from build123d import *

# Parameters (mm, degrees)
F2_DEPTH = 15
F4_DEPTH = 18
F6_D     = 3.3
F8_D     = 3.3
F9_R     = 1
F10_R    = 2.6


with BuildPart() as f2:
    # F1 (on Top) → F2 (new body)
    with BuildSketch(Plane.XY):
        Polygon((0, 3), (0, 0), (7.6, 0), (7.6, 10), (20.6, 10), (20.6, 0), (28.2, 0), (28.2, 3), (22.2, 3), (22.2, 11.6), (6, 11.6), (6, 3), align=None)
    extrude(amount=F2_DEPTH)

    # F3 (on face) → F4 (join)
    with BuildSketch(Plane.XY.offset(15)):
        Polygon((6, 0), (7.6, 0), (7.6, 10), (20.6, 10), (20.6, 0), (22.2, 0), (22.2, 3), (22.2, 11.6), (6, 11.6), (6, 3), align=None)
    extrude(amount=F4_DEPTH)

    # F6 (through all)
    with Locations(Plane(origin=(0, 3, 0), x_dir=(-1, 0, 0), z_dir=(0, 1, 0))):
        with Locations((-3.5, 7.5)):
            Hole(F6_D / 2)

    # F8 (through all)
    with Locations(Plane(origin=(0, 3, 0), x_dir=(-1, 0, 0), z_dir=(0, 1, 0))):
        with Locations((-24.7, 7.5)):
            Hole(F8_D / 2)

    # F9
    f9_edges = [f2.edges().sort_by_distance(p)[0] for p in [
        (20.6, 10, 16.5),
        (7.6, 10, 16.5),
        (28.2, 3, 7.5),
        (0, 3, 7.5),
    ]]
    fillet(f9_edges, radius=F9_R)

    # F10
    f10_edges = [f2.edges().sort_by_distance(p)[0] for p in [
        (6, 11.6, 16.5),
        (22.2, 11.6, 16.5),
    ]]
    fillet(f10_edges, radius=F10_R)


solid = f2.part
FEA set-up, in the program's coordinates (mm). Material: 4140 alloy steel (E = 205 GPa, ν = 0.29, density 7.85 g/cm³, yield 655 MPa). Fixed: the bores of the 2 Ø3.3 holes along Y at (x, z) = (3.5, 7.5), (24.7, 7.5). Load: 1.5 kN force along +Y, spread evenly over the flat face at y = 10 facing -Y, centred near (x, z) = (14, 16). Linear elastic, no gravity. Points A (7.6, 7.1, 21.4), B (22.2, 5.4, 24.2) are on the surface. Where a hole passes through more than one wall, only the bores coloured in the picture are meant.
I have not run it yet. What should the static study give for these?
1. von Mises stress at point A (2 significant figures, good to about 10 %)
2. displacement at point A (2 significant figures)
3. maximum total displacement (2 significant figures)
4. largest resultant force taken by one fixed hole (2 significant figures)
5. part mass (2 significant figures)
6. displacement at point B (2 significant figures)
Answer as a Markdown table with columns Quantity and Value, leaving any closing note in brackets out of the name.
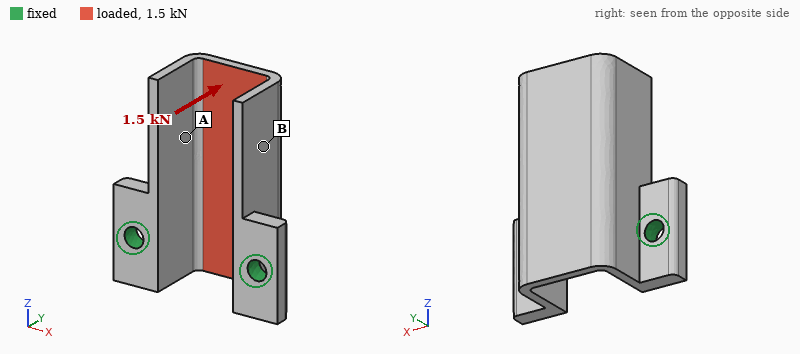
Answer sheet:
| Quantity | Value |
|---|---|
| von Mises stress at point A | 98 MPa |
| displacement at point A | 0.044 mm |
| maximum total displacement | 0.10 mm |
| largest resultant force taken by one fixed hole | 800 N |
| part mass | 18 g |
| displacement at point B | 0.049 mm |
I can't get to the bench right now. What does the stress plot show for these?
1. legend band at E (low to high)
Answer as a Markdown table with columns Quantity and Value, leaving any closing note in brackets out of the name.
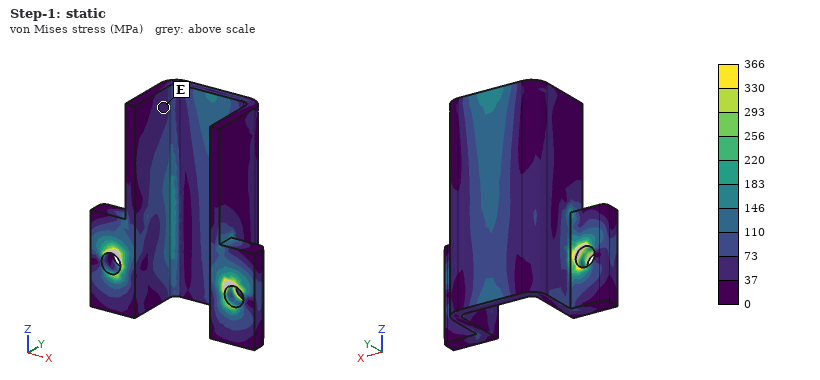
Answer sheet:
| Quantity | Value |
|---|---|
| legend band at E | 37 to 73 MPa |
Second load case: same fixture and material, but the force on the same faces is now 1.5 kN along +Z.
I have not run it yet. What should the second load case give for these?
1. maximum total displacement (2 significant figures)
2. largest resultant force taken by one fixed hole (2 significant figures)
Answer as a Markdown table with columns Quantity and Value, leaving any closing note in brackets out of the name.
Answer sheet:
| Quantity | Value |
|---|---|
| maximum total displacement | 69 µm |
| largest resultant force taken by one fixed hole | 750 N |
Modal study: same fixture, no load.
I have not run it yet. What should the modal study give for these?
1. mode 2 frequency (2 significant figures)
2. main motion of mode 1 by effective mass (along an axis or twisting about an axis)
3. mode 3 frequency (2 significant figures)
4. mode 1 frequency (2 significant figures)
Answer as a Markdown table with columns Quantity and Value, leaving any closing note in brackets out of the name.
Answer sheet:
| Quantity | Value |
|---|---|
| mode 2 frequency | 6200 Hz |
| main motion of mode 1 by effective mass | along X |
| mode 3 frequency | 10 kHz |
| mode 1 frequency | 5700 Hz |
